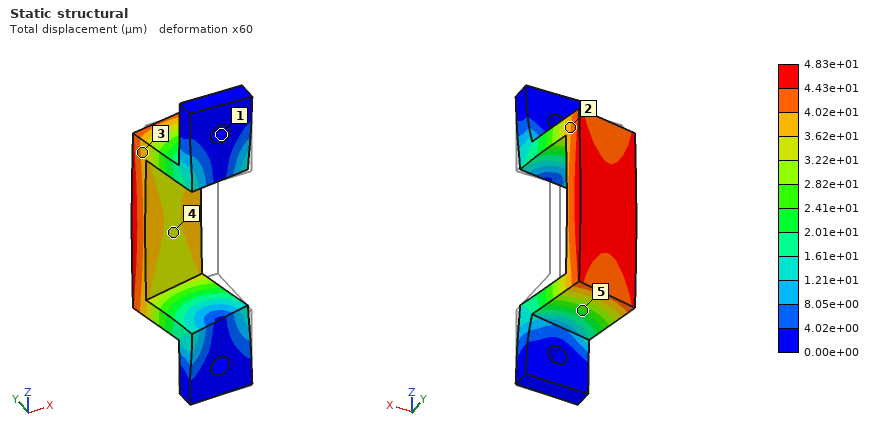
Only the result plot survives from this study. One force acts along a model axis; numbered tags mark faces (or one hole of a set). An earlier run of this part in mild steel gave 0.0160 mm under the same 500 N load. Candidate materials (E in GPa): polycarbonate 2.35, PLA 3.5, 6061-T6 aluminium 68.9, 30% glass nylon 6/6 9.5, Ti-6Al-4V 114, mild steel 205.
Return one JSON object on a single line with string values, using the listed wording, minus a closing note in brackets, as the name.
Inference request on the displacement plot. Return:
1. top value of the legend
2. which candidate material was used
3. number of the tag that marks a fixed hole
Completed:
{"top value of the legend": "4.83e+01 µm", "which candidate material was used": "6061-T6 aluminium", "number of the tag that marks a fixed hole": "1"}
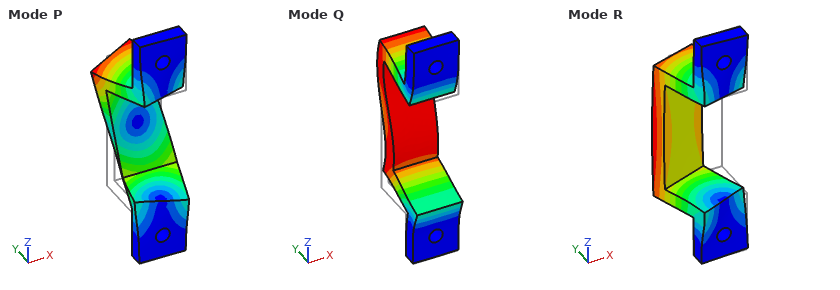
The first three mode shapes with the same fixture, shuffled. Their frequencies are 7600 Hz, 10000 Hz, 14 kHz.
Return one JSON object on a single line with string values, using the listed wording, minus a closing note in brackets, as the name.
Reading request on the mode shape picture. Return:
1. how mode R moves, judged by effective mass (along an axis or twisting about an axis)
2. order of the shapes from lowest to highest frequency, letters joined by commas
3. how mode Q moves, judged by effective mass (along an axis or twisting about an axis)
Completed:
{"how mode R moves, judged by effective mass": "along X", "order of the shapes from lowest to highest frequency, letters joined by commas": "R, Q, P", "how mode Q moves, judged by effective mass": "along Z"}
